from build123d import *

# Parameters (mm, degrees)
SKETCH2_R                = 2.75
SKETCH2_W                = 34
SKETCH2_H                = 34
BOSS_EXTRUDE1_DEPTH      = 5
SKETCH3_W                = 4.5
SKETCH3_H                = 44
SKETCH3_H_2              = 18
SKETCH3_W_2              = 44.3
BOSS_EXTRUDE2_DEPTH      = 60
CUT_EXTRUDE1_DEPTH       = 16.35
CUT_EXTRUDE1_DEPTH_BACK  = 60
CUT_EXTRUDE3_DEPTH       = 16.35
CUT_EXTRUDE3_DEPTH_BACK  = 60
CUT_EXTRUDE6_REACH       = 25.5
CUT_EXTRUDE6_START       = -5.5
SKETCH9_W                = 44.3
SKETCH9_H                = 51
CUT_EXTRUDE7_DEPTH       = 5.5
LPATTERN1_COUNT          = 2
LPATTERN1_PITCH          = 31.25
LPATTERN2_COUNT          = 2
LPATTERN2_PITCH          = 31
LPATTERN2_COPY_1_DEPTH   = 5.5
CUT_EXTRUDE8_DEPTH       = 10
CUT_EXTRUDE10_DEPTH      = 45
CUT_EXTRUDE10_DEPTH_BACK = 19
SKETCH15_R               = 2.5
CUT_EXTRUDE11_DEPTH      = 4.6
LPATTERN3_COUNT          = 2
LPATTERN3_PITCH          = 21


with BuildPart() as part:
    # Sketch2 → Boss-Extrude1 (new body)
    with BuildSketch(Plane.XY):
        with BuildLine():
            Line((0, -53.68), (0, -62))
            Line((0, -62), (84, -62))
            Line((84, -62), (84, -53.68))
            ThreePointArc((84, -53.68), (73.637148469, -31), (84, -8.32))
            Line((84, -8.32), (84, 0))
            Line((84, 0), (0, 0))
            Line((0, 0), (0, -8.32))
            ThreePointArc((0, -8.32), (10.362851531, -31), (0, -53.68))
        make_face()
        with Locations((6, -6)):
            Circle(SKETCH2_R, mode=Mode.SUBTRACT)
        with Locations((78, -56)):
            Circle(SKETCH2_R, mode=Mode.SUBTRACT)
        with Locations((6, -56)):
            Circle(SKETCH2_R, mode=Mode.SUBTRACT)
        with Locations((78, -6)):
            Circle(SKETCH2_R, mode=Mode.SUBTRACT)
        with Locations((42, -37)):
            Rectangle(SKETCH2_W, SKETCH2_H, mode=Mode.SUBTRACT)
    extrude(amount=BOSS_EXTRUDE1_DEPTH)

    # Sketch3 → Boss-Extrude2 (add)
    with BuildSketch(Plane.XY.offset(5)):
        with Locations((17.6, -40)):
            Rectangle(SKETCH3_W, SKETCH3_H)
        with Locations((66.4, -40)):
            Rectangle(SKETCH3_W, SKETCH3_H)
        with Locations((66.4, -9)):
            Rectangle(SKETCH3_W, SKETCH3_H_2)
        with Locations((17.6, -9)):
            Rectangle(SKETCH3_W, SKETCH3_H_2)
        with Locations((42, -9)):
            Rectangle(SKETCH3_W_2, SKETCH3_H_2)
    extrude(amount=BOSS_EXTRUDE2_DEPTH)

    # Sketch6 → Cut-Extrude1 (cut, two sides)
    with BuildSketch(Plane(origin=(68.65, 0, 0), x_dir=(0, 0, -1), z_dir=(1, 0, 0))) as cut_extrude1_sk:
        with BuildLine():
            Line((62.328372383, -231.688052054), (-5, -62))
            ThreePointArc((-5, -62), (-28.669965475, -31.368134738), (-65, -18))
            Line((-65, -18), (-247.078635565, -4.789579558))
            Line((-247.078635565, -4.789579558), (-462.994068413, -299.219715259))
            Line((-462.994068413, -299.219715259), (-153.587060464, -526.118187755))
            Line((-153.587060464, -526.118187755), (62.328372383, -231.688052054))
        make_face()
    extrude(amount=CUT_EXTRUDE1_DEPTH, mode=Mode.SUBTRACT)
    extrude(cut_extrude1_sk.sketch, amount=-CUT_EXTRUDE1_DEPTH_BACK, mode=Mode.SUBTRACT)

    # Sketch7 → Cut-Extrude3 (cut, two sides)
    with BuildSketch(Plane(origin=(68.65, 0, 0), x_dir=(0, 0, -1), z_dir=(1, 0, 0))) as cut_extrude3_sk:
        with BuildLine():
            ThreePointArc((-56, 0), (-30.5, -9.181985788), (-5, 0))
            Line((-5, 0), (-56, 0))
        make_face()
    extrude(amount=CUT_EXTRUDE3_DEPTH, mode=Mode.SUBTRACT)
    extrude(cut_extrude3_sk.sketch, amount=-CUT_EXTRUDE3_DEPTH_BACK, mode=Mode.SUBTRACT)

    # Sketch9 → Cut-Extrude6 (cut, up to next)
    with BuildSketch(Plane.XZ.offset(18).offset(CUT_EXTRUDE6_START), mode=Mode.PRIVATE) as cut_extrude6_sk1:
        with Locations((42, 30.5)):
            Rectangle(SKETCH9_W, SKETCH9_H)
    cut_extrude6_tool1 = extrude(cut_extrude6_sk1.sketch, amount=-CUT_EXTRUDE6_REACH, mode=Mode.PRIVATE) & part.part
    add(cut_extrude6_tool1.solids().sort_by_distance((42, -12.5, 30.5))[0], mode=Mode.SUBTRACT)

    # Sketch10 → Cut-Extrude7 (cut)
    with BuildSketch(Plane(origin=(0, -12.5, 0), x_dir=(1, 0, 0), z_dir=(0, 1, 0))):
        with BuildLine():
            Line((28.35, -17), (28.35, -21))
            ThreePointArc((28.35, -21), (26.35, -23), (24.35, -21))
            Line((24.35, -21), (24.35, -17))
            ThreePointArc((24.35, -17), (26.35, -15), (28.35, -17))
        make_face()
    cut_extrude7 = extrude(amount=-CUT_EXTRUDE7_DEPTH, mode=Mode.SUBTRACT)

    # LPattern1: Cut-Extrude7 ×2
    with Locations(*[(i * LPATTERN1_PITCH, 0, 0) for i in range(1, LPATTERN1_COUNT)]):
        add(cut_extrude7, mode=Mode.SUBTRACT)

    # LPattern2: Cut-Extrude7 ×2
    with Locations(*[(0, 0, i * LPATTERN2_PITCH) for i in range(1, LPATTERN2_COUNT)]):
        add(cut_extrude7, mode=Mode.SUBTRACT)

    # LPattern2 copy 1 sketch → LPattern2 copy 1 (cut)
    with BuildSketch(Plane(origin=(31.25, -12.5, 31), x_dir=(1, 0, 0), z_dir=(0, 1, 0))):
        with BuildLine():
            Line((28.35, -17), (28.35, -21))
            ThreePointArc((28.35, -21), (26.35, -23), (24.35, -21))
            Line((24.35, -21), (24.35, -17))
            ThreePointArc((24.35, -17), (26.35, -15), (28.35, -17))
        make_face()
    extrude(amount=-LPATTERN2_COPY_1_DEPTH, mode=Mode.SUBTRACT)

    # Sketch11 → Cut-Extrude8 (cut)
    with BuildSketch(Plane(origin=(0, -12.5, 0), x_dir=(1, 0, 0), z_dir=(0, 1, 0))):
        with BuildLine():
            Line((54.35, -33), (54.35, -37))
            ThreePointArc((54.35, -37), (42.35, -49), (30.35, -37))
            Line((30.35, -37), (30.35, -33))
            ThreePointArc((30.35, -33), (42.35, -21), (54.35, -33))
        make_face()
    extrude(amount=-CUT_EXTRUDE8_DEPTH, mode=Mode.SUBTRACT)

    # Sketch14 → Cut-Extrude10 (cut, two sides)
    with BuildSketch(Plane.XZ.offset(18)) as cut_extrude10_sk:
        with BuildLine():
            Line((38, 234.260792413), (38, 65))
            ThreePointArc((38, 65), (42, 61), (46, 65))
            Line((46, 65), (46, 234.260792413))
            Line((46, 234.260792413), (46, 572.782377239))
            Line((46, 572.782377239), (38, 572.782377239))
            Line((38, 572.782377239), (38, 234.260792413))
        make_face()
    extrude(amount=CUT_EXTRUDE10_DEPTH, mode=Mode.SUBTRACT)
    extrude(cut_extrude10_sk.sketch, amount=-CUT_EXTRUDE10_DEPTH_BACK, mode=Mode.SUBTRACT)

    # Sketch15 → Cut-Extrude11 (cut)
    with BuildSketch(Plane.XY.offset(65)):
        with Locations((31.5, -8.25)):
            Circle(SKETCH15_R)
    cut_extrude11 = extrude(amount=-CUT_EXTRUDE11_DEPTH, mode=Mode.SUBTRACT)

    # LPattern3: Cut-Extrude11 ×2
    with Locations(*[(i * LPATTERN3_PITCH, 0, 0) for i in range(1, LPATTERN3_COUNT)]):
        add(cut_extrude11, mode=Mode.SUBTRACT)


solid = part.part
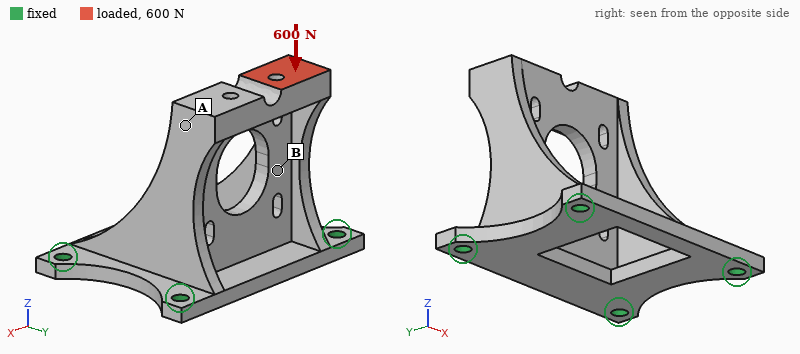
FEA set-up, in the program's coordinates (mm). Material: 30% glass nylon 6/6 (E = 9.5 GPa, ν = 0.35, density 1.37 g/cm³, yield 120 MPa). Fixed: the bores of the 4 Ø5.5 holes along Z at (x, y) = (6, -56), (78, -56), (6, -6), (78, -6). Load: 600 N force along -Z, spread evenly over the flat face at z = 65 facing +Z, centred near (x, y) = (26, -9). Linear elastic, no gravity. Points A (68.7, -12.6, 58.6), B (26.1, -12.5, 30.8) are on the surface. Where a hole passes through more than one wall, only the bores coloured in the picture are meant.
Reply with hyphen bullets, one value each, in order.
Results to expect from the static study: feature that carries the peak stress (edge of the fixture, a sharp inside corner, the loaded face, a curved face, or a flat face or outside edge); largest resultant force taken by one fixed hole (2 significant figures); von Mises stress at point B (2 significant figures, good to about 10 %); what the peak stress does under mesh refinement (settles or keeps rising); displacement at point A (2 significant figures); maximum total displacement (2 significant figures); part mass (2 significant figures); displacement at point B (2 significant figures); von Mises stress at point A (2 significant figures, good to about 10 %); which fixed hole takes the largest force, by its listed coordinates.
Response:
- edge of the fixture
- 430 N
- 6.9 MPa
- keeps rising
- 0.085 mm
- 0.26 mm
- 63 g
- 0.067 mm
- 2.6 MPa
- (6, -6)
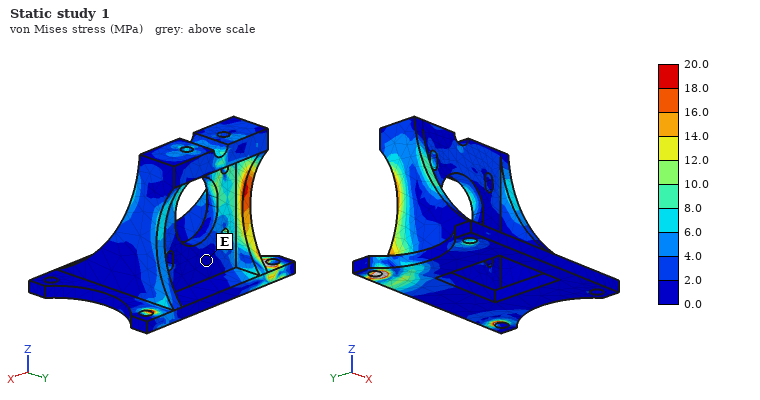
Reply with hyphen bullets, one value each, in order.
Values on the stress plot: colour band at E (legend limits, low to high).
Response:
- 0.0 to 2.0 MPa
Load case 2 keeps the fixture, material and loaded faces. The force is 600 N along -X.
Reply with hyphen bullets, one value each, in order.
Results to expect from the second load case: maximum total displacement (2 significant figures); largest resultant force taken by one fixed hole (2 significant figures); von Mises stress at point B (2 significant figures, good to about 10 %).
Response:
- 0.26 mm
- 520 N
- 7.7 MPa
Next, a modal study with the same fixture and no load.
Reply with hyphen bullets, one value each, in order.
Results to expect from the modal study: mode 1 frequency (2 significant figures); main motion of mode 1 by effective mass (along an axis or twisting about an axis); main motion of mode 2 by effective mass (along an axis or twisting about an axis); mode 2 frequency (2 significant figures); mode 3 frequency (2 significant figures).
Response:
- 1300 Hz
- along Y
- along X
- 1900 Hz
- 2300 Hz
